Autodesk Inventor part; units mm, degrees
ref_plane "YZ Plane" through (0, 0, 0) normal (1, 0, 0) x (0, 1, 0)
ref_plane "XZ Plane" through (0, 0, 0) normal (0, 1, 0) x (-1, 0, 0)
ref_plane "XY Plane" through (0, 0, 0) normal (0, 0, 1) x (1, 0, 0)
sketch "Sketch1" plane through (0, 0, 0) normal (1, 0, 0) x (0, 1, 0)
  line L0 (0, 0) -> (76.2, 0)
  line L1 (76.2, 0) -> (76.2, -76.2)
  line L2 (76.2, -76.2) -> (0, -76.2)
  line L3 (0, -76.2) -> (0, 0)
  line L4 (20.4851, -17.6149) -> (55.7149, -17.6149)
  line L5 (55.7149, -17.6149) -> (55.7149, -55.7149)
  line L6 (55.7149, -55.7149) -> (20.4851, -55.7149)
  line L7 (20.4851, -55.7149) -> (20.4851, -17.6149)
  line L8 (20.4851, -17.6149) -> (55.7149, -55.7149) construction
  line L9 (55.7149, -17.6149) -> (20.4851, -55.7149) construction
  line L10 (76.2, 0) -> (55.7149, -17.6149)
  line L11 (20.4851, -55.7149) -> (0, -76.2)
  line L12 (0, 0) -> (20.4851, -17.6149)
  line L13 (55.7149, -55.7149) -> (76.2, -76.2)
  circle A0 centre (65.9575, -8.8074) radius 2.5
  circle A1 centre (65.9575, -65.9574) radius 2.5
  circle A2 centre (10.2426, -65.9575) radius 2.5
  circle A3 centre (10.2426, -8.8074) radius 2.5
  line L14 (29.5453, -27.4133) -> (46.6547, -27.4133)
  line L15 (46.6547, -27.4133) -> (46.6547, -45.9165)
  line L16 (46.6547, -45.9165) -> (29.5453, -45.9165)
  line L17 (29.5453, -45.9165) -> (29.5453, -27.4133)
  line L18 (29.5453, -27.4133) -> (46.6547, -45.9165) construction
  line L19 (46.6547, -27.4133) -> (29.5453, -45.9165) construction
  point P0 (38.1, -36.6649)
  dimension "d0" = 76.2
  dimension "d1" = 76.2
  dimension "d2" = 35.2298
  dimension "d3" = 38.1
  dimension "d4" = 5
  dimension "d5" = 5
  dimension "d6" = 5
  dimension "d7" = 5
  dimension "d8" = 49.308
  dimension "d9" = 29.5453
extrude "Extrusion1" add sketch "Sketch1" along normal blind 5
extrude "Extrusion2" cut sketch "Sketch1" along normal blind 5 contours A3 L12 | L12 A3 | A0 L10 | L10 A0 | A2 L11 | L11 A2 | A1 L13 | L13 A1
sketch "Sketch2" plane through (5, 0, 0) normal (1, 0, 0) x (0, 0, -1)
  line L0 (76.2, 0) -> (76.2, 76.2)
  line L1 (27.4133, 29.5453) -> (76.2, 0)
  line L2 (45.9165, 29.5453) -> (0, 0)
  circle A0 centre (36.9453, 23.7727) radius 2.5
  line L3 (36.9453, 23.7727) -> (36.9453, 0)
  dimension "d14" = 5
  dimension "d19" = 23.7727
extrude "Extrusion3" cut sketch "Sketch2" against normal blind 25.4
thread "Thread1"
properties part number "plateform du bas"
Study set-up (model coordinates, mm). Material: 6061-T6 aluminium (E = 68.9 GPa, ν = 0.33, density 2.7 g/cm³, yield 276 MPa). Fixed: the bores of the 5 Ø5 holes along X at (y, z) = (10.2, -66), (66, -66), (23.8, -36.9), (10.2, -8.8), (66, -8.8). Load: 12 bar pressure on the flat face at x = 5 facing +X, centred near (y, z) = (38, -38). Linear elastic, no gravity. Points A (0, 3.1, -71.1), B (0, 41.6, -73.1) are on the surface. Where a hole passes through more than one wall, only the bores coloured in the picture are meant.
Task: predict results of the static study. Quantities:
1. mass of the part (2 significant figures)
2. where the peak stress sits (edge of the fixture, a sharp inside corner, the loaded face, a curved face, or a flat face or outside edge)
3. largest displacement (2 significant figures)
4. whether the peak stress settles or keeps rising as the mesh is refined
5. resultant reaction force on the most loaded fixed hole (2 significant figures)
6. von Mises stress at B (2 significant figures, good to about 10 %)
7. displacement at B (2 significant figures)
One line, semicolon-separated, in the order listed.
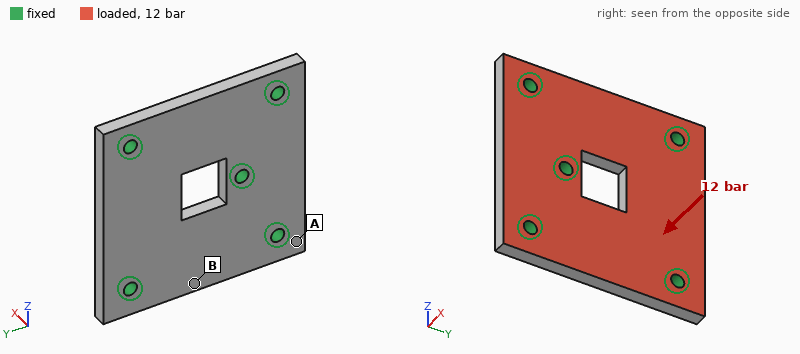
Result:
73 g; edge of the fixture; 61 µm; keeps rising; 1.5 kN; 32 MPa; 39 µm
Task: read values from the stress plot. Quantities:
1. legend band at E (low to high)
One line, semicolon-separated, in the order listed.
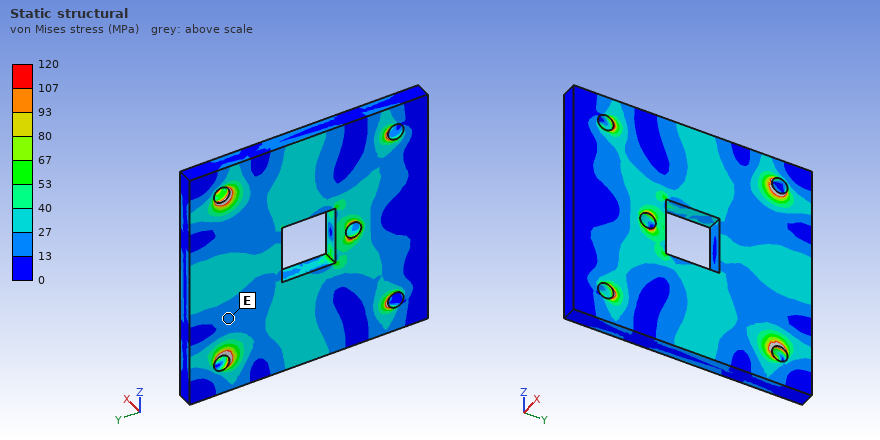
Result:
13 to 27 MPa
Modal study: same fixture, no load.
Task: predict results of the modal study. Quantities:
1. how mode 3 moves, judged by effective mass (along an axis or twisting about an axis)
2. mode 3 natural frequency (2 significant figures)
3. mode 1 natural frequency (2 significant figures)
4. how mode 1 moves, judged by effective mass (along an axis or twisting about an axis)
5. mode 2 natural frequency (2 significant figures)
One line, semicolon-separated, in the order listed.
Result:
twisting about Y; 9000 Hz; 7500 Hz; along X; 8700 Hz
